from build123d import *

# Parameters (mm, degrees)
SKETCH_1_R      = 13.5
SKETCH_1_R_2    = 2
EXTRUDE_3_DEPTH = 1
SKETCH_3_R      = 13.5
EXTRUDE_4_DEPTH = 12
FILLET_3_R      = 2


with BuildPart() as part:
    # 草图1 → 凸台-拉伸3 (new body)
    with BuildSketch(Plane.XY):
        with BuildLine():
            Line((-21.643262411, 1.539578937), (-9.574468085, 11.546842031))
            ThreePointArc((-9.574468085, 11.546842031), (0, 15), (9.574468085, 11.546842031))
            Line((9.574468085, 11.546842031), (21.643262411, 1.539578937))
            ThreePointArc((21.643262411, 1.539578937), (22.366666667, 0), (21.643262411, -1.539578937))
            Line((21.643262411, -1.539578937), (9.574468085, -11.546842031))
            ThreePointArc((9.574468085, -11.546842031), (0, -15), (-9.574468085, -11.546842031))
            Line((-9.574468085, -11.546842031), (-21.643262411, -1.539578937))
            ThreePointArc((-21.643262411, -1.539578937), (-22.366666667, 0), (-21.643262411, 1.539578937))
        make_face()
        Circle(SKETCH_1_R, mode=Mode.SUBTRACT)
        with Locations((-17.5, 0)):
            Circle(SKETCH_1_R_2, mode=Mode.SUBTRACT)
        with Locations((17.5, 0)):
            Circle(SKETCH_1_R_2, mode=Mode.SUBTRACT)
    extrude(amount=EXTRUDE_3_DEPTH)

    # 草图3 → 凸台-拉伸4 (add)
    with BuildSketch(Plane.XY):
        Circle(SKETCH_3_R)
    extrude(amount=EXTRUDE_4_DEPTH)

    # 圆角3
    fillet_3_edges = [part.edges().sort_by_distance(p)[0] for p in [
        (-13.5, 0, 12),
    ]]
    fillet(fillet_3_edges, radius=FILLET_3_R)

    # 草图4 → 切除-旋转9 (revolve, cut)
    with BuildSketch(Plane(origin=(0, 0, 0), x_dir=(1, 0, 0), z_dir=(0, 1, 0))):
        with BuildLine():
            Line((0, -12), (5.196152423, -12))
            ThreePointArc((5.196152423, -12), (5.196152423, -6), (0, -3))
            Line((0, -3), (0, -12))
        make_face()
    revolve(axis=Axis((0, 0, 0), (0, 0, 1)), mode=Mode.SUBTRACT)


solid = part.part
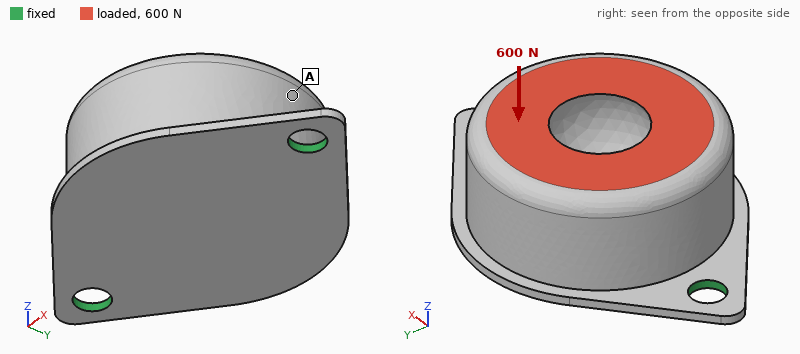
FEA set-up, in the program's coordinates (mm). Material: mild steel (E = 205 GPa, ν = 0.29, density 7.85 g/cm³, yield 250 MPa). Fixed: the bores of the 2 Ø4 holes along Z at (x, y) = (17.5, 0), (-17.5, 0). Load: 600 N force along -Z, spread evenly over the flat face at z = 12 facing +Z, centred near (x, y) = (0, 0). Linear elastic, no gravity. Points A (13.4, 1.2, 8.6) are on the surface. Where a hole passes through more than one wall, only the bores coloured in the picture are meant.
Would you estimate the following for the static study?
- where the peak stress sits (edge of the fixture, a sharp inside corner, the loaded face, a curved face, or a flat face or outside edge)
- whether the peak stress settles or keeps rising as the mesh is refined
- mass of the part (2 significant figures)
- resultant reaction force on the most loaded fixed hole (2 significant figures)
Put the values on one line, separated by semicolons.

edge of the fixture; keeps rising; 49 g; 360 N
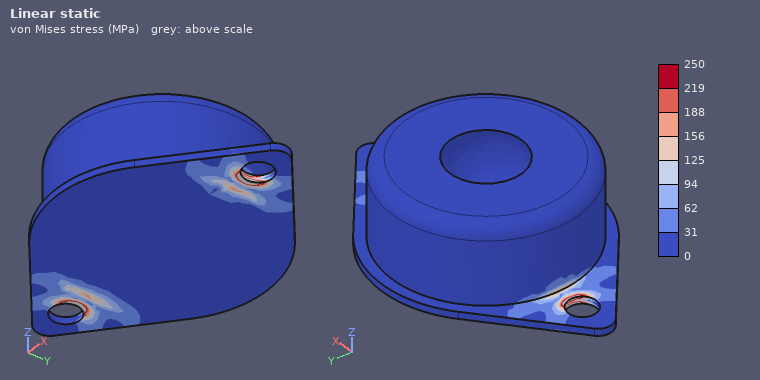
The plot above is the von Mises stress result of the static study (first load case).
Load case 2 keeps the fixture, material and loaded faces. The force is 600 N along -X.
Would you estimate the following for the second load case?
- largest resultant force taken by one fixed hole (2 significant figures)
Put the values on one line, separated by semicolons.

380 N
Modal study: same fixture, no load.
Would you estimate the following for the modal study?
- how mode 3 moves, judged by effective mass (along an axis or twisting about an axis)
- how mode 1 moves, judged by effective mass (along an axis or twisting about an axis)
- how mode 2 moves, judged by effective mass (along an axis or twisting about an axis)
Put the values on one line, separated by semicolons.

along X; along Y; along Z
